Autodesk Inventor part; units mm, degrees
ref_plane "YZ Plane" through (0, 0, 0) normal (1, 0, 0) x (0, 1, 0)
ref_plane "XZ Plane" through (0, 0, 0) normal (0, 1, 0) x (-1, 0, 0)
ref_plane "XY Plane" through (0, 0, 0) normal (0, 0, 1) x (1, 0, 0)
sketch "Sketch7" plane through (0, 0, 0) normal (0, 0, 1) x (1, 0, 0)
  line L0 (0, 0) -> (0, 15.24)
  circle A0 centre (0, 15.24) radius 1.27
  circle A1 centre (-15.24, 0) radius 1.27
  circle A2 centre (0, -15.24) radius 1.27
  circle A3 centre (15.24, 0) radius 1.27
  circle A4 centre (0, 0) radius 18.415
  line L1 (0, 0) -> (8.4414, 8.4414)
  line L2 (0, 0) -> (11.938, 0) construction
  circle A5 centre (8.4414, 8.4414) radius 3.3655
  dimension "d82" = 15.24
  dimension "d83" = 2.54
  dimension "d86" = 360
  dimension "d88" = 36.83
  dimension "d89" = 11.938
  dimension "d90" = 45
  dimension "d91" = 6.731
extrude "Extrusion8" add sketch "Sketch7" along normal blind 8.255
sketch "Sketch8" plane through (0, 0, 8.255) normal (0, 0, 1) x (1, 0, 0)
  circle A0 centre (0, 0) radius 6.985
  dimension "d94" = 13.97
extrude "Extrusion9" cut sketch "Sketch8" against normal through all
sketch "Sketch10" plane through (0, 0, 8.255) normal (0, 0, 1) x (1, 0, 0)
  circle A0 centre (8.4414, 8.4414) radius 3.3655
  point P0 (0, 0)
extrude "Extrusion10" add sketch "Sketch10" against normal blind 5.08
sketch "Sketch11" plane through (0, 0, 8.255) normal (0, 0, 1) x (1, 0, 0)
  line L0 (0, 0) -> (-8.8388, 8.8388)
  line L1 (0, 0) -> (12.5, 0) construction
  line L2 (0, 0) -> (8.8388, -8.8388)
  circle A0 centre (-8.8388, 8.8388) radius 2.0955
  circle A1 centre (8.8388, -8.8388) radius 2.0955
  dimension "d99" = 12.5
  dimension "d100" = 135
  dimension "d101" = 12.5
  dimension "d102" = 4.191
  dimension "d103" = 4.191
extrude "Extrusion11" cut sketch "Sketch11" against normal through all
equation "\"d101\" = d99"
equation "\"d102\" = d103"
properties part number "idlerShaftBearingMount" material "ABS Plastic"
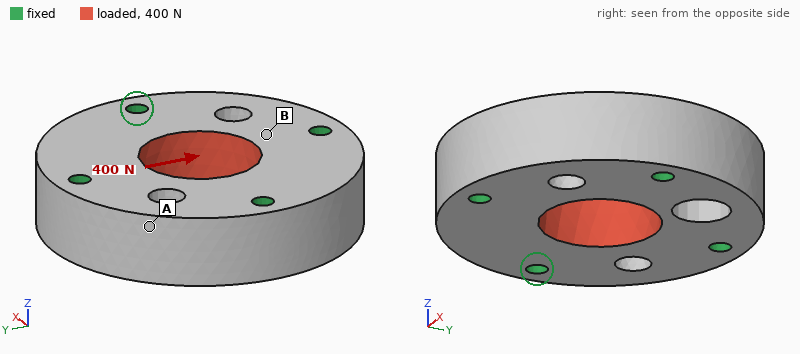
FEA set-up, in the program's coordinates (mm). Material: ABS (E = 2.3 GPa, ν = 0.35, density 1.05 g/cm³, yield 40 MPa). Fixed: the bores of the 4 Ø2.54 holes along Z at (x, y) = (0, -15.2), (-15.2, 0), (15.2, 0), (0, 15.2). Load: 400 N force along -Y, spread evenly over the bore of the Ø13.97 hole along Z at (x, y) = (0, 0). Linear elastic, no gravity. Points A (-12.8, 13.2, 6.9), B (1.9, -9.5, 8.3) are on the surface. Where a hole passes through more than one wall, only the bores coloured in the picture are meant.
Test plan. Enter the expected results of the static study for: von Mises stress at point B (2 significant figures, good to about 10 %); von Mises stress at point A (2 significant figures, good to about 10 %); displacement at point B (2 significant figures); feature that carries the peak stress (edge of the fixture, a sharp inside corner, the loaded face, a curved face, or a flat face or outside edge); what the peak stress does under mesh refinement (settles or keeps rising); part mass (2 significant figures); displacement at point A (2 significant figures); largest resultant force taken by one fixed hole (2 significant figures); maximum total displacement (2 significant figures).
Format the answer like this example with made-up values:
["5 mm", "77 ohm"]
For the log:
["1.6 MPa", "0.57 MPa", "4.6 µm", "edge of the fixture", "keeps rising", "7.4 g", "4.4 µm", "120 N", "12 µm"]
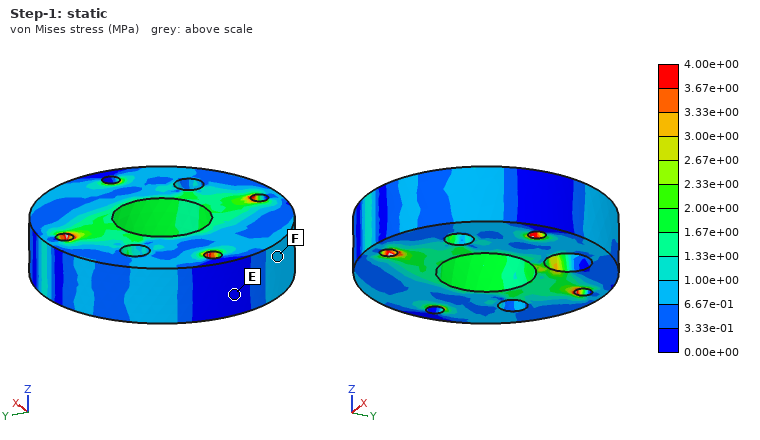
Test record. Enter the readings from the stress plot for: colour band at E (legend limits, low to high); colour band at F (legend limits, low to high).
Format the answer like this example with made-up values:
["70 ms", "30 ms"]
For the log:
["0.00e+00 to 3.33e-01 MPa", "6.67e-01 to 1.00e+00 MPa"]
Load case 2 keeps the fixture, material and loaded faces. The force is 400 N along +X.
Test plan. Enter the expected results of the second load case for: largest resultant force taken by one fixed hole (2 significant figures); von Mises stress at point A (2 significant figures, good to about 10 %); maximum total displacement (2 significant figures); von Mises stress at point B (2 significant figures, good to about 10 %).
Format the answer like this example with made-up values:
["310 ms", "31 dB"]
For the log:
["120 N", "0.60 MPa", "13 µm", "0.62 MPa"]
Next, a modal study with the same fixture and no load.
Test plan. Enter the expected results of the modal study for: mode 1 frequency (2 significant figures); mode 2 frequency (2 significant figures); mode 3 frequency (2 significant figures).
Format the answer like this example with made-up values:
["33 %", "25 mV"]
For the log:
["13 kHz", "14 kHz", "14 kHz"]
